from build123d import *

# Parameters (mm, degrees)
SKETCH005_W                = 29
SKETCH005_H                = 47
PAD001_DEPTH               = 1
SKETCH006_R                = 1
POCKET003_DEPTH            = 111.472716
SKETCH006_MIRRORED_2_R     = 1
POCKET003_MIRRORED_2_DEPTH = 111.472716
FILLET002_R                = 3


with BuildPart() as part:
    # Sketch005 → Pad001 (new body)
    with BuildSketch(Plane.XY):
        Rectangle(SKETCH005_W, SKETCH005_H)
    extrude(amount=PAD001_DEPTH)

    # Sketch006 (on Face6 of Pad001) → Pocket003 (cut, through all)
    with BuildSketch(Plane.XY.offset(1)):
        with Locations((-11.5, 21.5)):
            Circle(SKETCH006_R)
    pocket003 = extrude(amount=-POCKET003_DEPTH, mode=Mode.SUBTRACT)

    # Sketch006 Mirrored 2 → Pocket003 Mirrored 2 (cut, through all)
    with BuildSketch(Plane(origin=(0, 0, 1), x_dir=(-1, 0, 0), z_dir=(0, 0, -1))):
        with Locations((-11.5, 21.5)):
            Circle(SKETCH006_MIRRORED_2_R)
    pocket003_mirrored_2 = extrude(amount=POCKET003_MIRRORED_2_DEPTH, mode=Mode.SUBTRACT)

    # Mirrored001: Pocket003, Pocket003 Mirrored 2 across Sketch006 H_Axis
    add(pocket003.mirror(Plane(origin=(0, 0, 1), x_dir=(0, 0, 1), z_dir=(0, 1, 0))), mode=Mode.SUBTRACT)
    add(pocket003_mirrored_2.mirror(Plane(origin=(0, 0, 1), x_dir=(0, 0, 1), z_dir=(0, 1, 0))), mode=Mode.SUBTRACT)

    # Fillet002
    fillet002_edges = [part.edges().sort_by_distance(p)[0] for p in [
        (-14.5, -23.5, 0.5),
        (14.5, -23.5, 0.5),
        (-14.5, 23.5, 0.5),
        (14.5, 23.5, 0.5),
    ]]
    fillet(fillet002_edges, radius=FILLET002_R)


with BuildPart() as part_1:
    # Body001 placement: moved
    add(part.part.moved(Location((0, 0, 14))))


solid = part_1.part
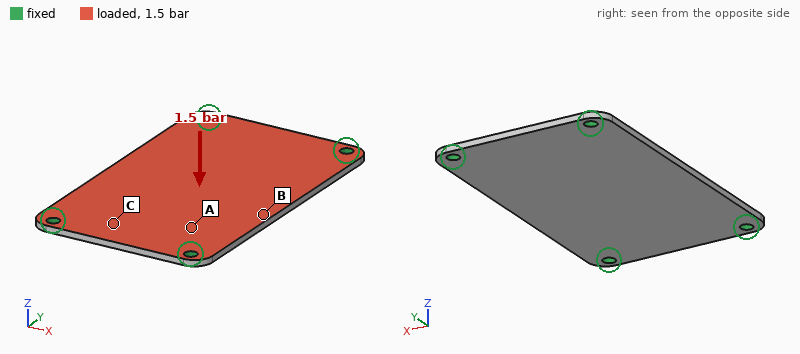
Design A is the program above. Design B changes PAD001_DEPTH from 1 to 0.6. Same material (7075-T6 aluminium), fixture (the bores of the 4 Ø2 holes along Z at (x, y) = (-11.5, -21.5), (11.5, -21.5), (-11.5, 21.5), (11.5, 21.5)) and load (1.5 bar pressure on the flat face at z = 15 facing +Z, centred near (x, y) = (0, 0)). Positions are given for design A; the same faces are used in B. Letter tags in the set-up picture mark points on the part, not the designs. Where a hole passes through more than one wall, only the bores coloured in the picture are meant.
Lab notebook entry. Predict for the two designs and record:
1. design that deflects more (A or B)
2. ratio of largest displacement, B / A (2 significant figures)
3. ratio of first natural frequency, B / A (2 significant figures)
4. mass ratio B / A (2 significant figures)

B
4.5
0.61
0.60
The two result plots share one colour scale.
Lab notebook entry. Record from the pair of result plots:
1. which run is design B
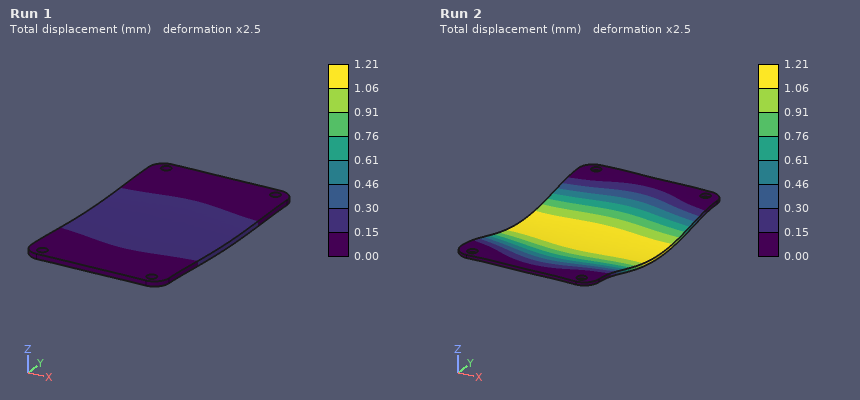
Run 2
